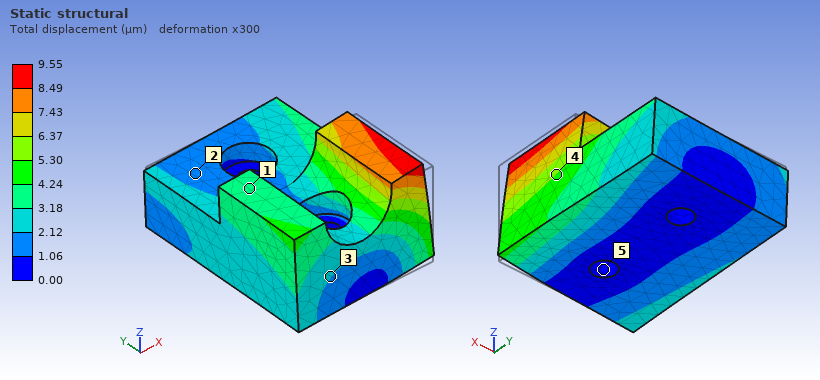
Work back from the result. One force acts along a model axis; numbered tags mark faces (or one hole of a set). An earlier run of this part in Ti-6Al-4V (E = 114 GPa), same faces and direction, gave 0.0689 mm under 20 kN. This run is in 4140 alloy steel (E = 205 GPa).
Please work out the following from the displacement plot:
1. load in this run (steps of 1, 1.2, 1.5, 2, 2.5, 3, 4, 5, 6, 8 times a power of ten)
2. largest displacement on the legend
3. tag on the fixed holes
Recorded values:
5 kN
9.55 µm
5
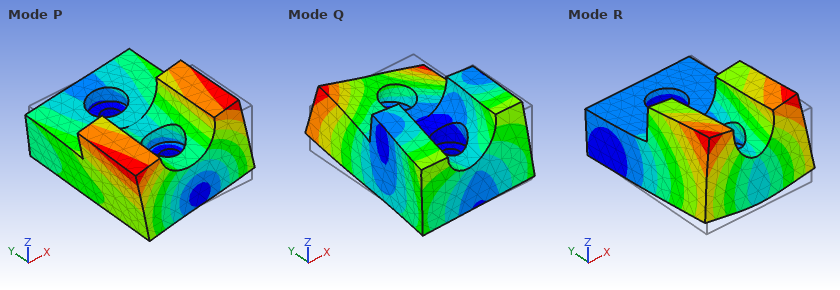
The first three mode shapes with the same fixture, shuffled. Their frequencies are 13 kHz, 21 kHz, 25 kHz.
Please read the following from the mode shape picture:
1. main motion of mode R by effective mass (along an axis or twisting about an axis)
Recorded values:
along Z
